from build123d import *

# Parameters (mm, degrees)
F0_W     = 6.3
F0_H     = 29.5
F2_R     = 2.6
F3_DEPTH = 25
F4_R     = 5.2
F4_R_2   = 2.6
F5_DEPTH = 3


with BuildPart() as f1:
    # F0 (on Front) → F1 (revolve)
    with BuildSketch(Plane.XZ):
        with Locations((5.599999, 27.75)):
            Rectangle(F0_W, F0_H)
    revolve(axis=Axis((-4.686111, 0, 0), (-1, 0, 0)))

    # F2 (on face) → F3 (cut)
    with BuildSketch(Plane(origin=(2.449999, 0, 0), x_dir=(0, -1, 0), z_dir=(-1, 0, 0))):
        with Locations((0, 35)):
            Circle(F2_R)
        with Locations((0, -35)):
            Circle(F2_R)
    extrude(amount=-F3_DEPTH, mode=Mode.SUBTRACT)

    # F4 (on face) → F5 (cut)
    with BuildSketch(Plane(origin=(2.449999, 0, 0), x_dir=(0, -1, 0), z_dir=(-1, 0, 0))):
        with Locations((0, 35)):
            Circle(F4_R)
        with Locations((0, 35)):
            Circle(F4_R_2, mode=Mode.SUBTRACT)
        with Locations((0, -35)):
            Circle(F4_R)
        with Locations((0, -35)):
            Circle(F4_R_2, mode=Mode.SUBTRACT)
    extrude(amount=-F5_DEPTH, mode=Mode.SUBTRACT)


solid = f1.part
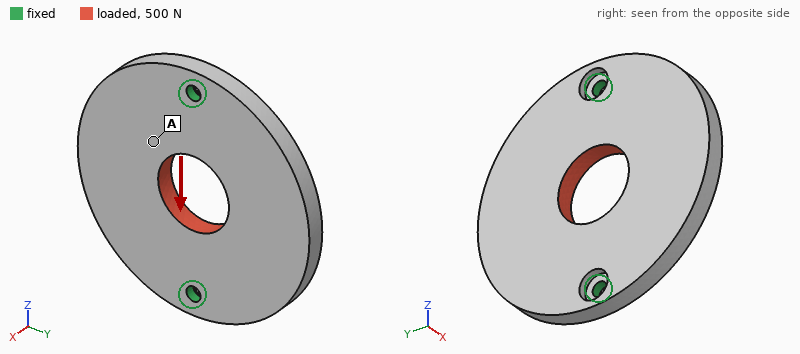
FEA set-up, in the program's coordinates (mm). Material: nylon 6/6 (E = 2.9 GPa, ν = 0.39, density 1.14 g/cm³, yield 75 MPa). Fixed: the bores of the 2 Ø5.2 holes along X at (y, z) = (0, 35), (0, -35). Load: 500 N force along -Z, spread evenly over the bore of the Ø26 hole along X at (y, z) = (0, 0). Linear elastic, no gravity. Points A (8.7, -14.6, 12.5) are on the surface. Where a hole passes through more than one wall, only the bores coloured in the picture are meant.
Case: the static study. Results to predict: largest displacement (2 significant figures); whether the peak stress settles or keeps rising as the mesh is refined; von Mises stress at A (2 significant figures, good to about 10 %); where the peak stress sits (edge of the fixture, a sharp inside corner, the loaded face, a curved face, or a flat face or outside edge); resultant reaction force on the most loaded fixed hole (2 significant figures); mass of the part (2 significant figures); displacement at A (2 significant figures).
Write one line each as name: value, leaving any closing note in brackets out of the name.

largest displacement: 27 µm
whether the peak stress settles or keeps rising as the mesh is refined: keeps rising
von Mises stress at A: 1.2 MPa
where the peak stress sits: edge of the fixture
resultant reaction force on the most loaded fixed hole: 250 N
mass of the part: 36 g
displacement at A: 22 µm
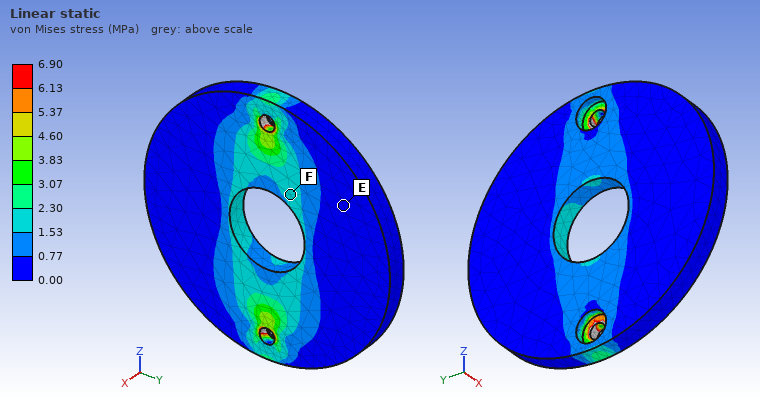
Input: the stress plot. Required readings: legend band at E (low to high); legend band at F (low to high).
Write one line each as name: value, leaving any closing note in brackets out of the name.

legend band at E: 0.00 to 0.77 MPa
legend band at F: 1.53 to 2.30 MPa
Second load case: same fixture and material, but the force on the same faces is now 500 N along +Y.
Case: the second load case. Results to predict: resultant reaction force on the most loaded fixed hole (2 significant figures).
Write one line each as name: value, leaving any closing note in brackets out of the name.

resultant reaction force on the most loaded fixed hole: 250 N
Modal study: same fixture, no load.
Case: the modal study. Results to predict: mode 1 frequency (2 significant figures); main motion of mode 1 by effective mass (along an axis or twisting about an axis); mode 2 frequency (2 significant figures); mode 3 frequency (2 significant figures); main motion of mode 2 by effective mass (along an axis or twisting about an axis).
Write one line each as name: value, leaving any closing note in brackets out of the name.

mode 1 frequency: 490 Hz
main motion of mode 1 by effective mass: twisting about Z
mode 2 frequency: 800 Hz
mode 3 frequency: 1700 Hz
main motion of mode 2 by effective mass: along X
